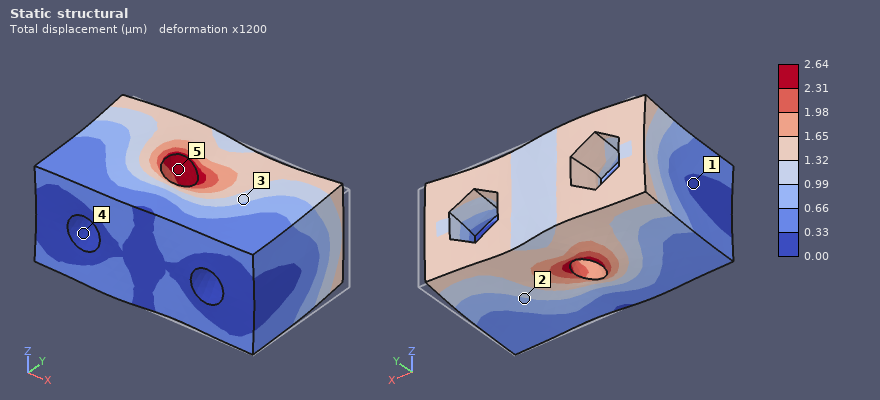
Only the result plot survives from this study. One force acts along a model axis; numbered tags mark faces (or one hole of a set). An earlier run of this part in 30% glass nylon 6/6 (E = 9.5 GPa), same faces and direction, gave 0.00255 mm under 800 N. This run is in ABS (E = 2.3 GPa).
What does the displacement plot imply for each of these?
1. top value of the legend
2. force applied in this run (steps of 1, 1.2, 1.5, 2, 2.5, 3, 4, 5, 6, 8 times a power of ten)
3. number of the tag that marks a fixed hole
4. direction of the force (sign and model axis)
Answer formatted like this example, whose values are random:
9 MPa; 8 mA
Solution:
2.64 µm; 200 N; 4; -X
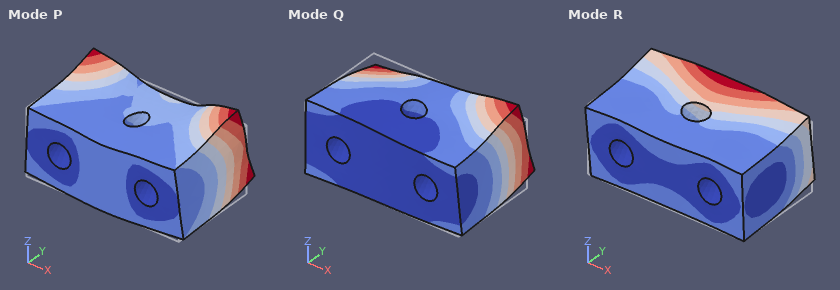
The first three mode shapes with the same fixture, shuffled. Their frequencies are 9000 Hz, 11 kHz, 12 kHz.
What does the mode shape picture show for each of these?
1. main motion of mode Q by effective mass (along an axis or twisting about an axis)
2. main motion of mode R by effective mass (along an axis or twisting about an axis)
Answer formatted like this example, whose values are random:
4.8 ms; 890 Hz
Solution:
twisting about Y; along Z
